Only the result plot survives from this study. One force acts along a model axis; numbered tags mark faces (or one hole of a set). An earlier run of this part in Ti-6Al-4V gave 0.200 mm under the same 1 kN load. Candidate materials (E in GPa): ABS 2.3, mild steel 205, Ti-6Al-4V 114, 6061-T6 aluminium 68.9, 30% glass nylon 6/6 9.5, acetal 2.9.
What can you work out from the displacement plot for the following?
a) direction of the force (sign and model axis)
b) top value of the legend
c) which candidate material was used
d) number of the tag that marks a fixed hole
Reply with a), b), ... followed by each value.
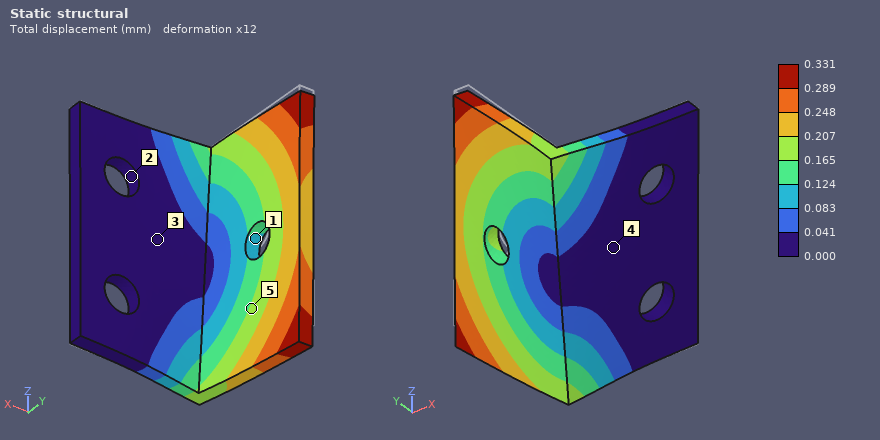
a) -Z
b) 0.331 mm
c) 6061-T6 aluminium
d) 2
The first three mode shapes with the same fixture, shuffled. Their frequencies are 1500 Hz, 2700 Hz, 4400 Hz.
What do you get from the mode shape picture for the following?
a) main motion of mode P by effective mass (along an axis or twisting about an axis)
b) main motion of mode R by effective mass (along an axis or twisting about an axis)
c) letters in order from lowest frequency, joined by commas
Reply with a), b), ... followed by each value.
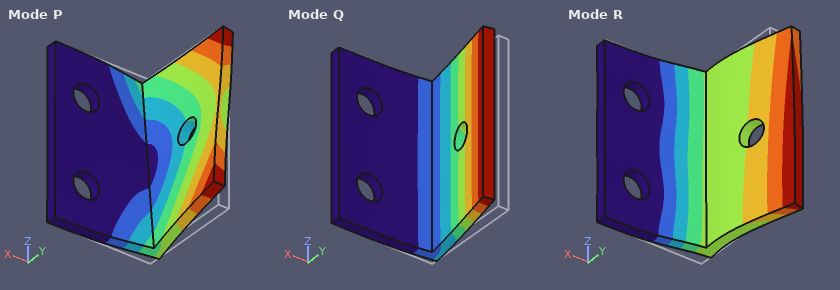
a) along Z
b) along Y
c) Q, P, R
